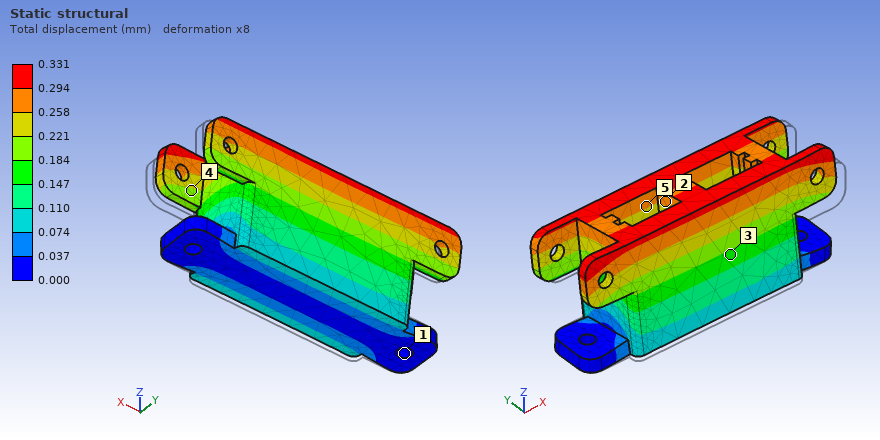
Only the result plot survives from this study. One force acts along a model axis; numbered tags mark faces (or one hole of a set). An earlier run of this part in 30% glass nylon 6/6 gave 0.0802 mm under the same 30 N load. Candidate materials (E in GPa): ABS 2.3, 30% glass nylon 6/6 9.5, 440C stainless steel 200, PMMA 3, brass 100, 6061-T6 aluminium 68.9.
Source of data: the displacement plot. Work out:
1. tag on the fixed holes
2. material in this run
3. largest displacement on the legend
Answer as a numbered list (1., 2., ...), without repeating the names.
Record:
1. 1
2. ABS
3. 0.331 mm
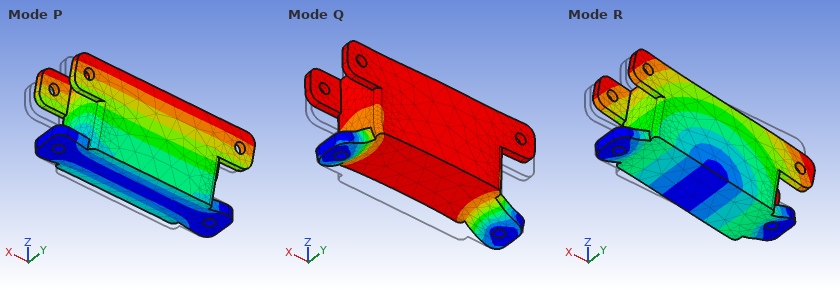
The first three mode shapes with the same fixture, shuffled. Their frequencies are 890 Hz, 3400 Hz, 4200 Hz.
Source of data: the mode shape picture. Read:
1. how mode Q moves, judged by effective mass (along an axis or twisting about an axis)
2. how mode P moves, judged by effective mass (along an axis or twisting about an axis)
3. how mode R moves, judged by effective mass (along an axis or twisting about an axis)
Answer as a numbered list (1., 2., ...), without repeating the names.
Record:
1. along Z
2. along Y
3. along X
